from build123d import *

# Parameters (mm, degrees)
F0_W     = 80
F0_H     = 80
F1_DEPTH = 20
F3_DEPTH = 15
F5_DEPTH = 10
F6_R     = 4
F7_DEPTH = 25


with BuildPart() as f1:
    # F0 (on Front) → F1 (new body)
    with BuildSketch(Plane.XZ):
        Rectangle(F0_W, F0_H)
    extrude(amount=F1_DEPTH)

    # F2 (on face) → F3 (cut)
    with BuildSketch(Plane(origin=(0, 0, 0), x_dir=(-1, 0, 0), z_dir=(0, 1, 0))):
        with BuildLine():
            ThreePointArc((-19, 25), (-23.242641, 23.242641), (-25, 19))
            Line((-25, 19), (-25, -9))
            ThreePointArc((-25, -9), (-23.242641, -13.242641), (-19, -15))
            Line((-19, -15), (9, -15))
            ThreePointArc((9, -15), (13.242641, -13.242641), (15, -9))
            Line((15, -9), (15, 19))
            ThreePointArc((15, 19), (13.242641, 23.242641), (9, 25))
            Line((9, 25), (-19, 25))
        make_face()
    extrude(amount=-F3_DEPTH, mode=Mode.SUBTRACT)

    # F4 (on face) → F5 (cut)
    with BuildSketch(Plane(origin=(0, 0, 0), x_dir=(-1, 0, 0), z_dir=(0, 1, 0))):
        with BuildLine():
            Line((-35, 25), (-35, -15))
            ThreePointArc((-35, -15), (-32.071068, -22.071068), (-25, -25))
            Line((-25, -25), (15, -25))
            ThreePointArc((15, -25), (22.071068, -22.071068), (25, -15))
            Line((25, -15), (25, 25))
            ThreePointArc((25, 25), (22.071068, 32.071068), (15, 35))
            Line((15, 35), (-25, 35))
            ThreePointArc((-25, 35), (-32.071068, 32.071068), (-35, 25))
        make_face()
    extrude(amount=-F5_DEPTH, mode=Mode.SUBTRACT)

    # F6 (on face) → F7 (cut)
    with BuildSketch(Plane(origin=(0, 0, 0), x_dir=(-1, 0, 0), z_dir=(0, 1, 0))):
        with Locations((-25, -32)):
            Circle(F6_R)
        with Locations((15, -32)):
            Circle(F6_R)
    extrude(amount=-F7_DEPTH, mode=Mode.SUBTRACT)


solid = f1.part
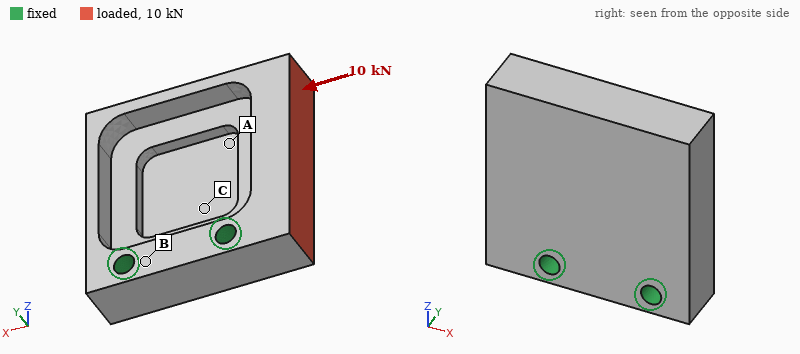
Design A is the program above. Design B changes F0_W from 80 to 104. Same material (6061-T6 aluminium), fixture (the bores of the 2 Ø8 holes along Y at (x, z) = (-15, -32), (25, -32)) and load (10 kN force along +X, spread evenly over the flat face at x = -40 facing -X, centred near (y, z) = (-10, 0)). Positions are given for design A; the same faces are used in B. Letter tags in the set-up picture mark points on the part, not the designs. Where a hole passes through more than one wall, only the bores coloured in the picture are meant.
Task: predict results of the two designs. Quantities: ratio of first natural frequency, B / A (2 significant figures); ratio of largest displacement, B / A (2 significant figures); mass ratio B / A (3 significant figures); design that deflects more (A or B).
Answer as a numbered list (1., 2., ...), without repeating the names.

1. 0.94
2. 0.85
3. 1.46
4. A
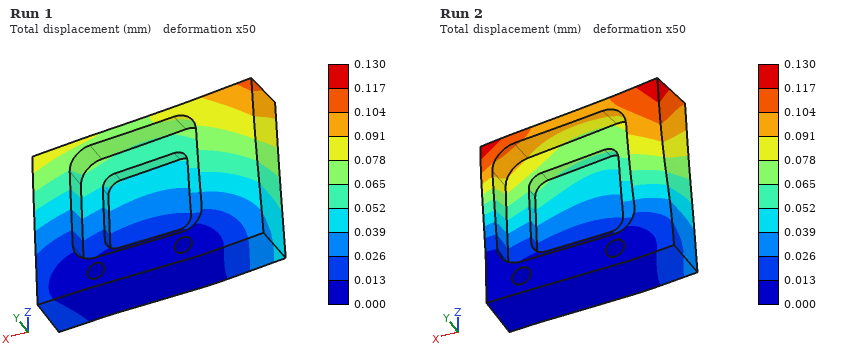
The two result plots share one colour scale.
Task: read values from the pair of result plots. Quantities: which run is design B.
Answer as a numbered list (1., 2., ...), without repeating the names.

1. Run 1
